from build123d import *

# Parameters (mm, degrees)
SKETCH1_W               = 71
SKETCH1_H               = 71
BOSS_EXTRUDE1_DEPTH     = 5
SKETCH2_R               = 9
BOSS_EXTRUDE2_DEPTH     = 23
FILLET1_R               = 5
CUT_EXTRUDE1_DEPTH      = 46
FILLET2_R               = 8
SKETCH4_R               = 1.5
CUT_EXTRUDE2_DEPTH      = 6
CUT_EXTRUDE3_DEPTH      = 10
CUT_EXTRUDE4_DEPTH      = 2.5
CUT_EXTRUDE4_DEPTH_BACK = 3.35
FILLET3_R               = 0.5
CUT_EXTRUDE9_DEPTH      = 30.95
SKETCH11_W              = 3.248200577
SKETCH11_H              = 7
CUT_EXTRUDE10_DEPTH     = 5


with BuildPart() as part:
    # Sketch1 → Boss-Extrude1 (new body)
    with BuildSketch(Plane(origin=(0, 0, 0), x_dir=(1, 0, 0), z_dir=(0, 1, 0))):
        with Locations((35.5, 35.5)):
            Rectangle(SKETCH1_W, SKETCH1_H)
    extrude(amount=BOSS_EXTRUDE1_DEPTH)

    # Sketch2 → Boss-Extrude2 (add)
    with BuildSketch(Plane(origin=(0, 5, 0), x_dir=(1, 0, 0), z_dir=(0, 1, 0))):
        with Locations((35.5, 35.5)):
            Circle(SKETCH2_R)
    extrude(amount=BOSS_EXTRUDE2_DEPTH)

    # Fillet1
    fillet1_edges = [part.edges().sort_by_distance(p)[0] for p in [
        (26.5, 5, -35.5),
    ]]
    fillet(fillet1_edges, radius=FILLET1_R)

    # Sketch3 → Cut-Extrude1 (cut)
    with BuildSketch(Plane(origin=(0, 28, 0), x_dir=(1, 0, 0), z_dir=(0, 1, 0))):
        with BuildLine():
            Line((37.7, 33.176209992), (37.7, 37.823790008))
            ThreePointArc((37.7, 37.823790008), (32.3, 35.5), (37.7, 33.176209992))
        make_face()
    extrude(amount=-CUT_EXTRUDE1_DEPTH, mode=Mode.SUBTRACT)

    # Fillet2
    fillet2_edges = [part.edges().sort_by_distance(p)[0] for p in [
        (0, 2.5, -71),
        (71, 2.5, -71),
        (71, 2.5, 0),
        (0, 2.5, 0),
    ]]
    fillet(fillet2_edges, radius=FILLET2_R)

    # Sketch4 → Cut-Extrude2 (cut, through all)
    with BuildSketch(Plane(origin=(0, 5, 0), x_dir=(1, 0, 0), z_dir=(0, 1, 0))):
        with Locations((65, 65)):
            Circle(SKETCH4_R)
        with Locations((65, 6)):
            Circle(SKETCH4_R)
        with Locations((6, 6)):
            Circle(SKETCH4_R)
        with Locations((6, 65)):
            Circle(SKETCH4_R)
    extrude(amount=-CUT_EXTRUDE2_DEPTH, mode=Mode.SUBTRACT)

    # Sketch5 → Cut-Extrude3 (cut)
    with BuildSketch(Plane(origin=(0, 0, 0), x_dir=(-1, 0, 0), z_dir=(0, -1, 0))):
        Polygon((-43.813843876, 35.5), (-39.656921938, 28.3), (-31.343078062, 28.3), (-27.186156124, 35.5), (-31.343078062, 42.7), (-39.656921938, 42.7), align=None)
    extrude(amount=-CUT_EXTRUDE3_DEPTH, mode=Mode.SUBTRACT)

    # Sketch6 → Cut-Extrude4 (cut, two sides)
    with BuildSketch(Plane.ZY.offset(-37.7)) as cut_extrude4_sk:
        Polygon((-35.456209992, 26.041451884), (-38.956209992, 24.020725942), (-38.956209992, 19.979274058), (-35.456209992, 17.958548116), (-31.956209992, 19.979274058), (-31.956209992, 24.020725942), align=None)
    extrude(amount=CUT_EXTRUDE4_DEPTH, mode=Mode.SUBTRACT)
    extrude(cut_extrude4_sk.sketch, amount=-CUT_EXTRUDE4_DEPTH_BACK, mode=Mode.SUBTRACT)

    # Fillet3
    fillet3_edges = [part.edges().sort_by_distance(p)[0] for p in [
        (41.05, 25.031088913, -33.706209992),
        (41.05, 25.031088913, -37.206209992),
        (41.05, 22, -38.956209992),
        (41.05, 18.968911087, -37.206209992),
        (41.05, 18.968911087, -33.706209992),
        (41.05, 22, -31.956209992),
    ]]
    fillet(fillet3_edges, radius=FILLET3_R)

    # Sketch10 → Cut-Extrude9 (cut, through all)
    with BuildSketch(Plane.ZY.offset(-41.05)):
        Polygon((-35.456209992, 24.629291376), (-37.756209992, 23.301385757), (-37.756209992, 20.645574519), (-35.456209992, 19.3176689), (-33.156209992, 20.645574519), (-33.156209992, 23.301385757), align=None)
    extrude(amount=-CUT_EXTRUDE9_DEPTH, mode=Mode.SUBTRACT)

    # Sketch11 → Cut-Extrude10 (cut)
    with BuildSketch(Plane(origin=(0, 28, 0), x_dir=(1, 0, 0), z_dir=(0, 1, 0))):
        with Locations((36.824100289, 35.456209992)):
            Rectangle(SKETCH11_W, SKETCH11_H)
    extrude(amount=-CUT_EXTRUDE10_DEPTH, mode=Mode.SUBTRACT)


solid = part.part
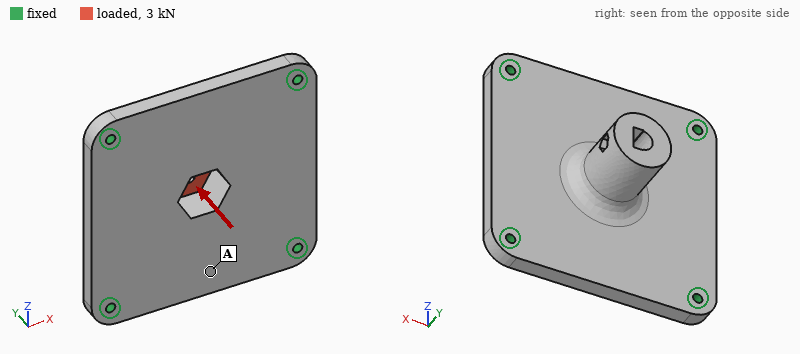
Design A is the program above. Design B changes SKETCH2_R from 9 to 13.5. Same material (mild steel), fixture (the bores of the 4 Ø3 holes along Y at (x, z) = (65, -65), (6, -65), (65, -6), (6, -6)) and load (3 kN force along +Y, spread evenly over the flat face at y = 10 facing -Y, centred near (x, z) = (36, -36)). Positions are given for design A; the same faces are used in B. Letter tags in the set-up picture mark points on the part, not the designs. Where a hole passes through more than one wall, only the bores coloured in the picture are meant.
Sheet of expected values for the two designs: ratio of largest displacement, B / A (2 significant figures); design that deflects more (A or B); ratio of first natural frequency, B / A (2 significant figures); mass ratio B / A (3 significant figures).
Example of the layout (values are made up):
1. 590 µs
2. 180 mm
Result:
1. 0.63
2. A
3. 0.93
4. 1.26
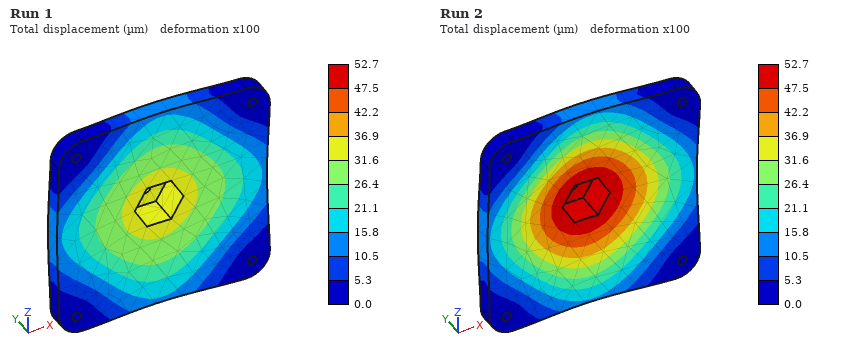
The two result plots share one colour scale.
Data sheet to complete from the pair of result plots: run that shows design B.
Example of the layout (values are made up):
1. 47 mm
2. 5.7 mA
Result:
1. Run 1
